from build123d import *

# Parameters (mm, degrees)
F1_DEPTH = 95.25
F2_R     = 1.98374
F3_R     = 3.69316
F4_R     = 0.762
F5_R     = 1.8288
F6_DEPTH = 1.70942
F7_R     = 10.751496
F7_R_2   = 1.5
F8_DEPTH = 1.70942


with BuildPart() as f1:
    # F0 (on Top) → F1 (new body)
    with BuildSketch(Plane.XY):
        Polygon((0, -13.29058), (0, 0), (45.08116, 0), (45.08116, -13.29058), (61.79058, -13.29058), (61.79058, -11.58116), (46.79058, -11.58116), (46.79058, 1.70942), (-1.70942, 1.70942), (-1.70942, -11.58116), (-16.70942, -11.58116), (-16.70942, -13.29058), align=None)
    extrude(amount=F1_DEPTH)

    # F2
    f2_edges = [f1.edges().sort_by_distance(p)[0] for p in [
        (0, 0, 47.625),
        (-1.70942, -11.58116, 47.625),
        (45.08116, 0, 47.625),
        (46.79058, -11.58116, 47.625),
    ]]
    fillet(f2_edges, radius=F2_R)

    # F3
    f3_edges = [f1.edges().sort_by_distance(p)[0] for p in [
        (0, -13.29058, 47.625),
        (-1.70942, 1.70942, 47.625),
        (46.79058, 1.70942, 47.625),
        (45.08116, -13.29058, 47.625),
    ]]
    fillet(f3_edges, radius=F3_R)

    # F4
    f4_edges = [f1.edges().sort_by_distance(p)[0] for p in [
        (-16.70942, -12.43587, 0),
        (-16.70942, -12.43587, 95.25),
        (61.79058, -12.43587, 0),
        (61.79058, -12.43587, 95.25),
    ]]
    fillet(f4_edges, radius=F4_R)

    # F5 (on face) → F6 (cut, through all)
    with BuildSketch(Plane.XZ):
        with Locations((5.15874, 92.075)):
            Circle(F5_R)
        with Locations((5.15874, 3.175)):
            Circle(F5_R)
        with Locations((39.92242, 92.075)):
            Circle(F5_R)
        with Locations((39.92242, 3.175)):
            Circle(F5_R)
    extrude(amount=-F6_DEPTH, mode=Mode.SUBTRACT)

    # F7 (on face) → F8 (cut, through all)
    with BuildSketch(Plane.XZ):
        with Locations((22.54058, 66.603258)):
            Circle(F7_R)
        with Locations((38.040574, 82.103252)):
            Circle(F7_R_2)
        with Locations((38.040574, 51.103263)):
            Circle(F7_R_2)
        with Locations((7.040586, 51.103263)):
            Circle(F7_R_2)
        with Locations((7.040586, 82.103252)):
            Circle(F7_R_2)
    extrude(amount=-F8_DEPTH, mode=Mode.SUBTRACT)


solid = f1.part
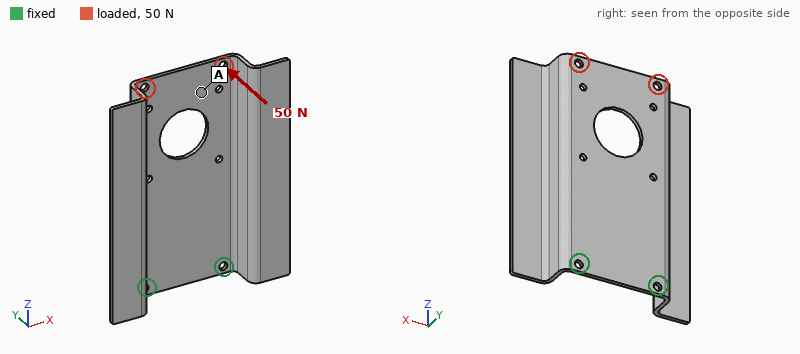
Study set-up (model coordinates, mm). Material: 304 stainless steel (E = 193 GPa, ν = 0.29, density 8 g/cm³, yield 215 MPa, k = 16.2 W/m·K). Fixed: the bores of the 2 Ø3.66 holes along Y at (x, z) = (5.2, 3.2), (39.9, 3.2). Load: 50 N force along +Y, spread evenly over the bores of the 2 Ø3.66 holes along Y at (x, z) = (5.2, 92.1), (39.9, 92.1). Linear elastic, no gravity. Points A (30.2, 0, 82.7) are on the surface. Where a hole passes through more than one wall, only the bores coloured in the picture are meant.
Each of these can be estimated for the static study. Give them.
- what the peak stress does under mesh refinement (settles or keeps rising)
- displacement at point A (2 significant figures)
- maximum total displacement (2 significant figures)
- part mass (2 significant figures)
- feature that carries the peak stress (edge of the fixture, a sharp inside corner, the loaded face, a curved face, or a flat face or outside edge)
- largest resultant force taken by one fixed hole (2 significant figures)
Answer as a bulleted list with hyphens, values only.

- keeps rising
- 0.35 mm
- 0.41 mm
- 120 g
- edge of the fixture
- 83 N
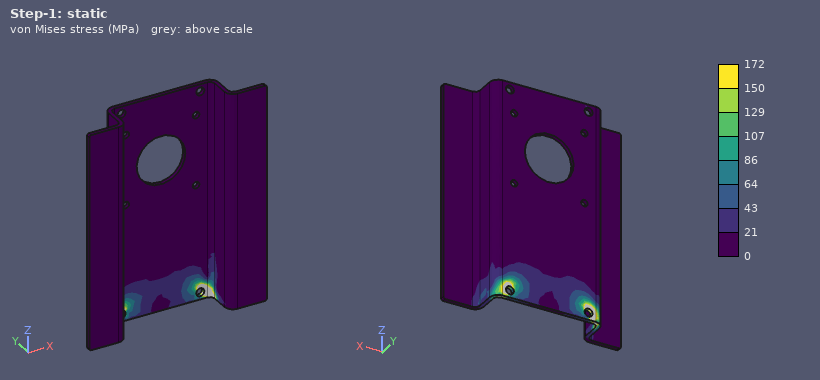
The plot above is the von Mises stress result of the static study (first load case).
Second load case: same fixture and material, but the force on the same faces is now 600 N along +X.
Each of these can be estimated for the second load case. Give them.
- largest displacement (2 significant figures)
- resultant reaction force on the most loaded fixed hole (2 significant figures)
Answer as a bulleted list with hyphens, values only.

- 84 µm
- 1.5 kN
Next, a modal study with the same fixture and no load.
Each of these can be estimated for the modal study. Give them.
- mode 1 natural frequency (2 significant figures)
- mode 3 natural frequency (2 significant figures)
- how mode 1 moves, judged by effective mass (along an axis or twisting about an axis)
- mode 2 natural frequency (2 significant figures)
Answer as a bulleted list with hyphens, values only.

- 280 Hz
- 1000 Hz
- along Y
- 380 Hz
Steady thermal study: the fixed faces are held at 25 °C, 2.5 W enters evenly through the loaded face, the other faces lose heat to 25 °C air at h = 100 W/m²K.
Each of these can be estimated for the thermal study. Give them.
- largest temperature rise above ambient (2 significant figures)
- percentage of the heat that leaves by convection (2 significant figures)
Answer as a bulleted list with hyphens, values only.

- 26 K
- 100 %
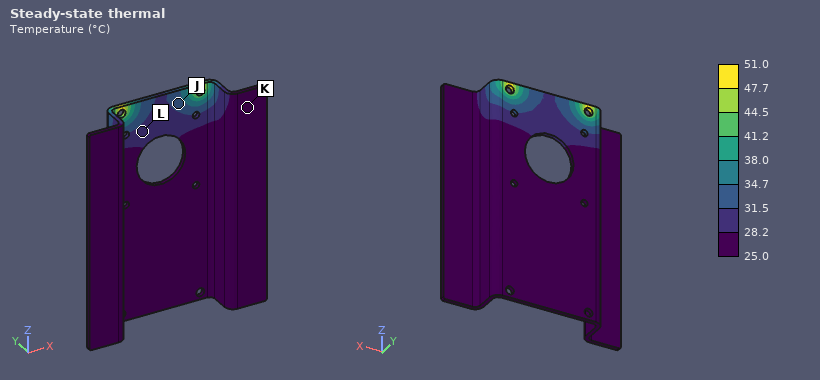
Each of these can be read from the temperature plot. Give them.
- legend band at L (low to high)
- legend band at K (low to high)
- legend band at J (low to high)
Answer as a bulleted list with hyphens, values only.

- 28.2 to 31.5 °C
- 25.0 to 28.2 °C
- 31.5 to 34.7 °C
